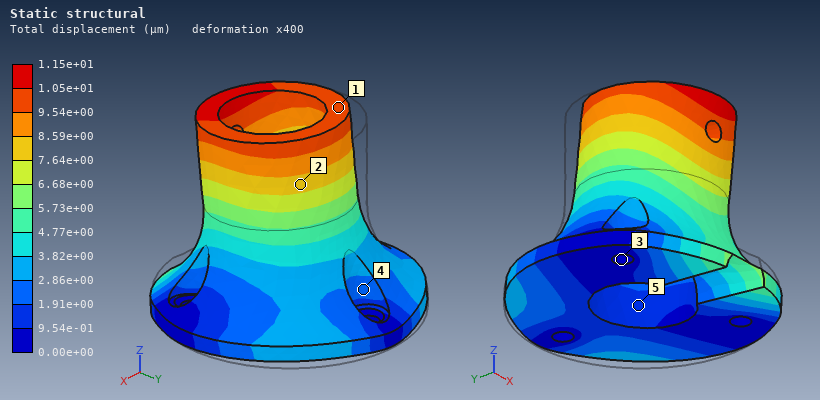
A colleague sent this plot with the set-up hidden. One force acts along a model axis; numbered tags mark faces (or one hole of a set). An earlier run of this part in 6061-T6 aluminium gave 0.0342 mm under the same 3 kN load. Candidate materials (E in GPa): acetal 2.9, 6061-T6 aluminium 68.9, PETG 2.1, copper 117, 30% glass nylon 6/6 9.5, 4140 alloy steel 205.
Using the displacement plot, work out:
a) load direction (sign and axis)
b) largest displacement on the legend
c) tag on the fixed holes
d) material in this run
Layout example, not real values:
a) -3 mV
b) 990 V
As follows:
a) -Y
b) 1.15e+01 µm
c) 3
d) 4140 alloy steel
